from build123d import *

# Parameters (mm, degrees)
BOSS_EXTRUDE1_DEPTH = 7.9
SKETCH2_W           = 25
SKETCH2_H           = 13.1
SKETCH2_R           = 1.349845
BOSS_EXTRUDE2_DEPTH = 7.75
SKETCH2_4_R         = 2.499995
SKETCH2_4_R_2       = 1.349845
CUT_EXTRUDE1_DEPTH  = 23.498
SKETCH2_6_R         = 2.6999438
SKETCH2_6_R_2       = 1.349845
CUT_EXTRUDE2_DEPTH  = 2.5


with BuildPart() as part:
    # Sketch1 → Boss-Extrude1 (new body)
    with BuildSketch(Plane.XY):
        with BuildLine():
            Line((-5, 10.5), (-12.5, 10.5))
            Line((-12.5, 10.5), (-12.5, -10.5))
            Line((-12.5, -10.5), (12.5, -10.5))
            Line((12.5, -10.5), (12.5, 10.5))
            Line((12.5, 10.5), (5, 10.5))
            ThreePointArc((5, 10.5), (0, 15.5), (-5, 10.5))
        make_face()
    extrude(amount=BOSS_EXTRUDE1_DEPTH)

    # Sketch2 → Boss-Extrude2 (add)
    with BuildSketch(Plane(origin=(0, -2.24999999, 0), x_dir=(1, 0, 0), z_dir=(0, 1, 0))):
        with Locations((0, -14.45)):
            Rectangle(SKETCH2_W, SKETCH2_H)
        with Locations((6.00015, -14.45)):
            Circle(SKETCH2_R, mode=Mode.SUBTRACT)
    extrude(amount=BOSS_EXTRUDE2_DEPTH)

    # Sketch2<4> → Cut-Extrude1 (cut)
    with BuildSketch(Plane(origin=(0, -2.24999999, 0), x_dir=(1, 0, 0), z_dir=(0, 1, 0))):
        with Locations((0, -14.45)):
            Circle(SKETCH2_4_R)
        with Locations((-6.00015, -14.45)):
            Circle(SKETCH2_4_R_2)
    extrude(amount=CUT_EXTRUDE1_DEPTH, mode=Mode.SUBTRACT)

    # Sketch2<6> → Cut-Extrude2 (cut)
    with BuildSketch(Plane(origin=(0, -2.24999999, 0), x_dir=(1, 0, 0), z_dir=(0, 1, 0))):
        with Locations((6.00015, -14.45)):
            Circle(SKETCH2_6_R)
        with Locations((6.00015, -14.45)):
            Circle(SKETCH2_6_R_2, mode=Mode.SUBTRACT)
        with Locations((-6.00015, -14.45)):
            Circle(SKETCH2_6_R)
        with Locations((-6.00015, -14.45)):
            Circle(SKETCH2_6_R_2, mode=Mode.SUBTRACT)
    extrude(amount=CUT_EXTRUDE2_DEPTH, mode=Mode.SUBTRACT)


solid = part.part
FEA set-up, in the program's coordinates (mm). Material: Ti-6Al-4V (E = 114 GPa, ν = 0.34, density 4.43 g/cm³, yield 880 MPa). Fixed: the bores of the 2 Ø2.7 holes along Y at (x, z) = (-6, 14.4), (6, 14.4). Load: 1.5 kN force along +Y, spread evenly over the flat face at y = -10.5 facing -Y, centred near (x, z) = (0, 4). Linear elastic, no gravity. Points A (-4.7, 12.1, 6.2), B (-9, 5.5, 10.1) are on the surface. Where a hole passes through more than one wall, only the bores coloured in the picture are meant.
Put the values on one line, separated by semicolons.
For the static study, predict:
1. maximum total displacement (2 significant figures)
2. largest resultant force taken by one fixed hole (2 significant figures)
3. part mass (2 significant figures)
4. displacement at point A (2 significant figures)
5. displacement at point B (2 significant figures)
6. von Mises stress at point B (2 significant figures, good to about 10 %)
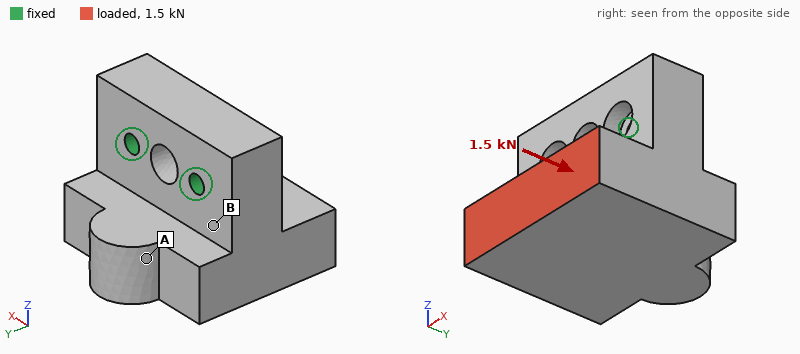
33 µm; 750 N; 30 g; 21 µm; 7.1 µm; 44 MPa
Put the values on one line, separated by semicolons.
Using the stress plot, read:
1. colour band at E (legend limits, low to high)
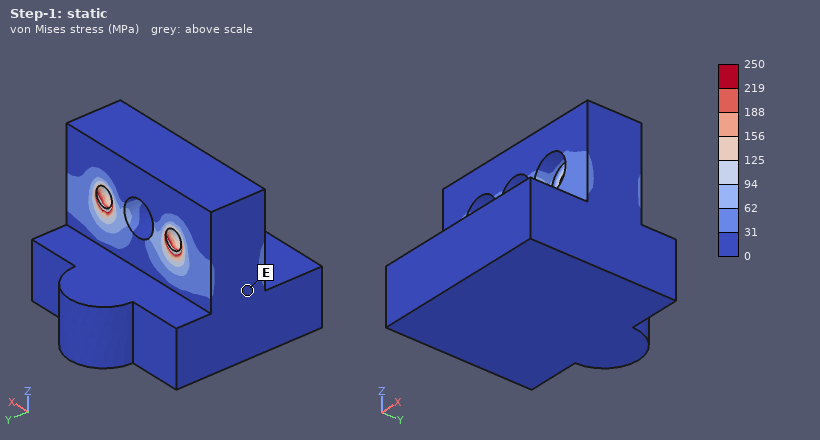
0 to 31 MPa
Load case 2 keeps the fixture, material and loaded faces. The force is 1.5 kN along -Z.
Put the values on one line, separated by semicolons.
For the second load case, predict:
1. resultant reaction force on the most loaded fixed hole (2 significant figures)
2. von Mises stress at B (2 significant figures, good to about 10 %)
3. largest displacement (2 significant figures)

760 N; 81 MPa; 57 µm
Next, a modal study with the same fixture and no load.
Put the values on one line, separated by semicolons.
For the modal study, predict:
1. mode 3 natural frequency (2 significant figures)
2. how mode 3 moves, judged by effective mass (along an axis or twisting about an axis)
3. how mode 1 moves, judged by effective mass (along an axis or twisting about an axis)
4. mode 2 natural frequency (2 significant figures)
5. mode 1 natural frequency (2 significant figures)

19 kHz; along X; along Y; 16 kHz; 8300 Hz
